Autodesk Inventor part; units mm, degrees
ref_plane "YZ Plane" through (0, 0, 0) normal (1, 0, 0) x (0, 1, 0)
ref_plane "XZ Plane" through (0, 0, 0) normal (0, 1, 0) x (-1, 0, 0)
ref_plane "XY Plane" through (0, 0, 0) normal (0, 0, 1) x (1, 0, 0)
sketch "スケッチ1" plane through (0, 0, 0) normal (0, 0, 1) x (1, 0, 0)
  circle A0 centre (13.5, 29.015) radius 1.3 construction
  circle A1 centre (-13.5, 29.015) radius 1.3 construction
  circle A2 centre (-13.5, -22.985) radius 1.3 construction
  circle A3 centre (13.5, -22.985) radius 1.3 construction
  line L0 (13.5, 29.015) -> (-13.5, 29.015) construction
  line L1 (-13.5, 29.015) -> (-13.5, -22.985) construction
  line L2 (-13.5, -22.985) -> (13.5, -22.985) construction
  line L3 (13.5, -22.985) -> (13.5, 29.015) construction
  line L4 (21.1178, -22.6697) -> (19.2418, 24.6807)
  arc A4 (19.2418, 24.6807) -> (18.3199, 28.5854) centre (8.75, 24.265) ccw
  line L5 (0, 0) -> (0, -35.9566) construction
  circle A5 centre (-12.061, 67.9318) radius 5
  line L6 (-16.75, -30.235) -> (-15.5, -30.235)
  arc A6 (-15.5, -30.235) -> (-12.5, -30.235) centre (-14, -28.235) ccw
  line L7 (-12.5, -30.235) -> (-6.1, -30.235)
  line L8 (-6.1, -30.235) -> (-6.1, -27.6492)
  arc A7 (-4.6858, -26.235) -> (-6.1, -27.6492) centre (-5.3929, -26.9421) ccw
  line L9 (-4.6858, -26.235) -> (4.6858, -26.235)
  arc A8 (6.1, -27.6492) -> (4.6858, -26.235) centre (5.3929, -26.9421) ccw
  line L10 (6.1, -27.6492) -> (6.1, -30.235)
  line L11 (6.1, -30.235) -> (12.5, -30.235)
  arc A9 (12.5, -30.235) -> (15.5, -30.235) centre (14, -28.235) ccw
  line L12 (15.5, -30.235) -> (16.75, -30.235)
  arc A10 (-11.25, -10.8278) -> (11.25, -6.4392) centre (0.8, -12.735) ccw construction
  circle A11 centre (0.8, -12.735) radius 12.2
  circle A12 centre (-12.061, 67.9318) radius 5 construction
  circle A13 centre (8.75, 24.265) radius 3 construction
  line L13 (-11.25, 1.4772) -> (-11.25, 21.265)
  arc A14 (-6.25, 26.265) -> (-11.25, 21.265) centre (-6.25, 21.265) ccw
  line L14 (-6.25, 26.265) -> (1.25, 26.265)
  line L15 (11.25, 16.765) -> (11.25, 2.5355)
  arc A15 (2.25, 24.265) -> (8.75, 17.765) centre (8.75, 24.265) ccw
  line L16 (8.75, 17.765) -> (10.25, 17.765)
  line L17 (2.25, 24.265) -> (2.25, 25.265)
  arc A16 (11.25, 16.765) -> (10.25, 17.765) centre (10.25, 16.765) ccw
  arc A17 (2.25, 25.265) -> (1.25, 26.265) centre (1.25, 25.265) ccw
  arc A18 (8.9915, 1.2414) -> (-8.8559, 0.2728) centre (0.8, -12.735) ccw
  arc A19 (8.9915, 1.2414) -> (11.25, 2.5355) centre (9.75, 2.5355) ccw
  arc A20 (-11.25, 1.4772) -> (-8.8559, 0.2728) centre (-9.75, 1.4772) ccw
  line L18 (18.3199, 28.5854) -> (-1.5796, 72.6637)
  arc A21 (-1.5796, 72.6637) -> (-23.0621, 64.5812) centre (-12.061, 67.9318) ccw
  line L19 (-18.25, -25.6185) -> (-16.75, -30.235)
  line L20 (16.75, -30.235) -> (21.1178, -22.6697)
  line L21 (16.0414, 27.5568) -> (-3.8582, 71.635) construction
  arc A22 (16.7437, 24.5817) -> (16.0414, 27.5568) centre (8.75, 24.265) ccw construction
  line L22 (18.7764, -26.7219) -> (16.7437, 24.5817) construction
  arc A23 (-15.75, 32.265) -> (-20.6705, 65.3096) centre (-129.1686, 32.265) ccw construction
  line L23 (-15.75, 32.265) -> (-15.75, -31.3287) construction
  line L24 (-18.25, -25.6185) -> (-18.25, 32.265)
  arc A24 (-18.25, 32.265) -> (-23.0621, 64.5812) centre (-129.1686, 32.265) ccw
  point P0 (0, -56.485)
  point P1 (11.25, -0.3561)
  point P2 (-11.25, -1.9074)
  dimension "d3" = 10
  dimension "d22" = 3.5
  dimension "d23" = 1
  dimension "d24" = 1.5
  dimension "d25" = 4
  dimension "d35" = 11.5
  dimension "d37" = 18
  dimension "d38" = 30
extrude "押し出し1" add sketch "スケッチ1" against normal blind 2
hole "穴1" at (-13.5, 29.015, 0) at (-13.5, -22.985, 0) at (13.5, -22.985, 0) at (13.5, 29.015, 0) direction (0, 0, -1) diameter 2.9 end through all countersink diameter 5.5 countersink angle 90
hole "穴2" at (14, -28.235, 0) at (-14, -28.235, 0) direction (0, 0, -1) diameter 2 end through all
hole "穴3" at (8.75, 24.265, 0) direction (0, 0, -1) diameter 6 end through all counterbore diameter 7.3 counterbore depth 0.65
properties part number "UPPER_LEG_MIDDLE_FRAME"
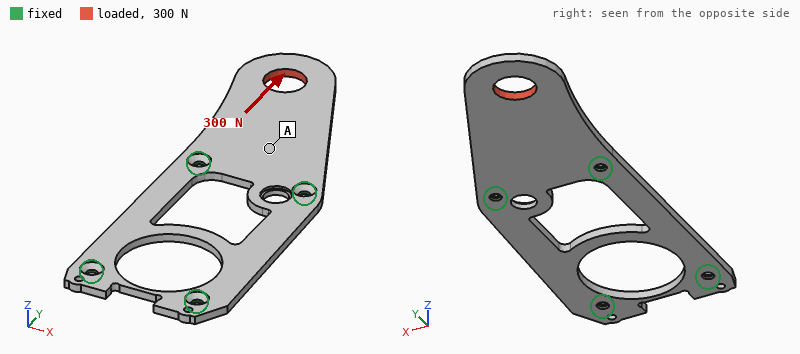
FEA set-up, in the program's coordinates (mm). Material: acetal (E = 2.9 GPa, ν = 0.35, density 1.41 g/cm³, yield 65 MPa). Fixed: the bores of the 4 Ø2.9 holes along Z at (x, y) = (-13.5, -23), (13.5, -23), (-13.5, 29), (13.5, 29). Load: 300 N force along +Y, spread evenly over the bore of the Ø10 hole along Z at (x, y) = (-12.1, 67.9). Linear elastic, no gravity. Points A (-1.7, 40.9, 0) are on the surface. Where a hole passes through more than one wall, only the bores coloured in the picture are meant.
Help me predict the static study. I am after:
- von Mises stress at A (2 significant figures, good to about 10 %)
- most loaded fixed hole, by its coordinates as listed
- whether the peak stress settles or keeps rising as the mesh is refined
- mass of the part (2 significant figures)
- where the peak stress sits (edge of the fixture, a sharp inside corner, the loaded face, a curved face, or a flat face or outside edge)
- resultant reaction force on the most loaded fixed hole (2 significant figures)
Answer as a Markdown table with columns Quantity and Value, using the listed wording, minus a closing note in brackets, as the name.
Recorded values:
| Quantity | Value |
|---|---|
| von Mises stress at A | 2.5 MPa |
| most loaded fixed hole, by its coordinates as listed | (-13.5, 29) |
| whether the peak stress settles or keeps rising as the mesh is refined | keeps rising |
| mass of the part | 6.9 g |
| where the peak stress sits | edge of the fixture |
| resultant reaction force on the most loaded fixed hole | 260 N |
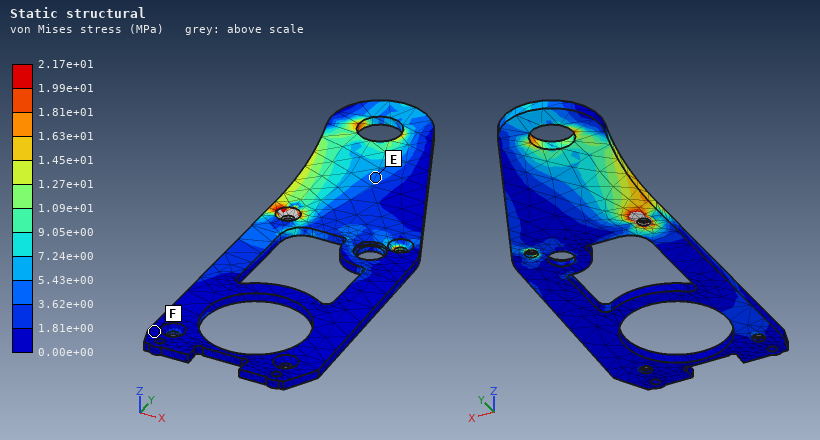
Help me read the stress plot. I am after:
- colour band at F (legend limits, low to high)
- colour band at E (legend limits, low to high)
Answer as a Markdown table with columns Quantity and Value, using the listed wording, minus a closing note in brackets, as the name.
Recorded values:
| Quantity | Value |
|---|---|
| colour band at F | 0.00e+00 to 1.81e+00 MPa |
| colour band at E | 3.62e+00 to 5.43e+00 MPa |
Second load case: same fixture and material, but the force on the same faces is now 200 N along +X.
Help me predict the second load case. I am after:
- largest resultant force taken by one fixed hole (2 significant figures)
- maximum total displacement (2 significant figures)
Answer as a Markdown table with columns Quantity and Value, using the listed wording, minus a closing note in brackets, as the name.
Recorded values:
| Quantity | Value |
|---|---|
| largest resultant force taken by one fixed hole | 300 N |
| maximum total displacement | 0.80 mm |
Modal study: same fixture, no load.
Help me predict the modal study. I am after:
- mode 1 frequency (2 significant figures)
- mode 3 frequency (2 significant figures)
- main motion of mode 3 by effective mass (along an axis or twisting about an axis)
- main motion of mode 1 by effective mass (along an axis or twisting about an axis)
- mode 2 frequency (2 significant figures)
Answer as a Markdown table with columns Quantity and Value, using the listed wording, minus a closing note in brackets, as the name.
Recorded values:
| Quantity | Value |
|---|---|
| mode 1 frequency | 200 Hz |
| mode 3 frequency | 900 Hz |
| main motion of mode 3 by effective mass | along Z |
| main motion of mode 1 by effective mass | along Z |
| mode 2 frequency | 840 Hz |
